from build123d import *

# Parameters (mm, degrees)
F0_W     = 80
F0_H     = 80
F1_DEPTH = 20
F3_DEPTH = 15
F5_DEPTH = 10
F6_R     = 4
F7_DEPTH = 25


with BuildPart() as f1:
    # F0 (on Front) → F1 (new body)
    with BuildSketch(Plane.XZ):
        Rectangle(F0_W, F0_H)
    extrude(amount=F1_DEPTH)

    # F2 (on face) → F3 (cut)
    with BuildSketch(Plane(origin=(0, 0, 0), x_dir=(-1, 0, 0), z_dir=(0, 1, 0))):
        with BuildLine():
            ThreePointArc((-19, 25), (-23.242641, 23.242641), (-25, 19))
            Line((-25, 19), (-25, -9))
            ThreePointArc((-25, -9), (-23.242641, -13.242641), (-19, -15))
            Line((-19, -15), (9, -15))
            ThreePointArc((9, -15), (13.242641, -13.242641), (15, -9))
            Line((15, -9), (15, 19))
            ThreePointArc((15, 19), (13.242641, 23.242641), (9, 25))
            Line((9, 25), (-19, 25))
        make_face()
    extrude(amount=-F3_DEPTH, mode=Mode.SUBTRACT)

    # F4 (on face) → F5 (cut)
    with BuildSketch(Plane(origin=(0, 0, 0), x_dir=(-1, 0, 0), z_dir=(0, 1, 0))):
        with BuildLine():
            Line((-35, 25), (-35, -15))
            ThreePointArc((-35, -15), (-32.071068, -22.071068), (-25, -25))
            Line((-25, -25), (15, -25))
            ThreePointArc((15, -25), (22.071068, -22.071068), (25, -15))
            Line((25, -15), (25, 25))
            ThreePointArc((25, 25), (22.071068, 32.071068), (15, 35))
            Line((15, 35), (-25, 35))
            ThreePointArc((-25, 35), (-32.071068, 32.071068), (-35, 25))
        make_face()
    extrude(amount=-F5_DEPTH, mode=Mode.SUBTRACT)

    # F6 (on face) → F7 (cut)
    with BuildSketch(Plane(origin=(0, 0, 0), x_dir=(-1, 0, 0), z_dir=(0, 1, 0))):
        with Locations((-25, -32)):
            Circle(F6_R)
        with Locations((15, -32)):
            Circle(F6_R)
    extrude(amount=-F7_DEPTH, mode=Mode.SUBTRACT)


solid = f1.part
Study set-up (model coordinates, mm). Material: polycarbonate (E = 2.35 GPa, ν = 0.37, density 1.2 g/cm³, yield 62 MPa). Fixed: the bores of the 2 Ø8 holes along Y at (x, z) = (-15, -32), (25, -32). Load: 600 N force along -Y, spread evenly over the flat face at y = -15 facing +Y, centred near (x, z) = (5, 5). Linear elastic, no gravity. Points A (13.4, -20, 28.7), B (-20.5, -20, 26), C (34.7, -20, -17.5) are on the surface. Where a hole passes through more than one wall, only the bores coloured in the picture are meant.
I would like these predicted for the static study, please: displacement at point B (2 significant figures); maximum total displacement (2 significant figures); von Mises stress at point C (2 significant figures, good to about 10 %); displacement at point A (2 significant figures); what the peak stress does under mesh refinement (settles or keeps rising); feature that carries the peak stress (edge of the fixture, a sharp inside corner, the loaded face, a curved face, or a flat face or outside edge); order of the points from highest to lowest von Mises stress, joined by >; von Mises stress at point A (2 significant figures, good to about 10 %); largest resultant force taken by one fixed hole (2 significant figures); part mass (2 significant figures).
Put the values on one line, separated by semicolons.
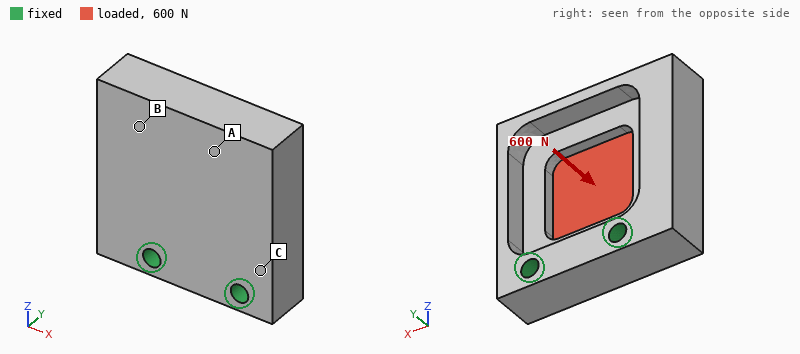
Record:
0.52 mm; 0.78 mm; 6.4 MPa; 0.66 mm; keeps rising; edge of the fixture; C > A > B; 3.6 MPa; 310 N; 100 g
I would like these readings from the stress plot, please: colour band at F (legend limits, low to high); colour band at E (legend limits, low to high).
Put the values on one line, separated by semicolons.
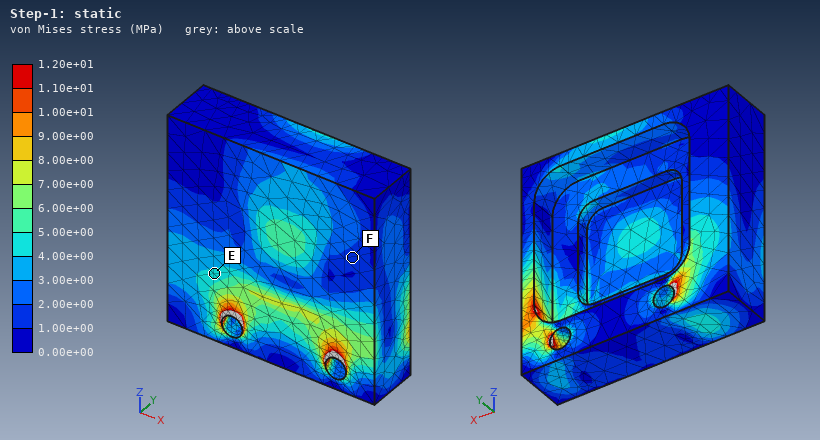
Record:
1.00e+00 to 2.00e+00 MPa; 4.00e+00 to 5.00e+00 MPa
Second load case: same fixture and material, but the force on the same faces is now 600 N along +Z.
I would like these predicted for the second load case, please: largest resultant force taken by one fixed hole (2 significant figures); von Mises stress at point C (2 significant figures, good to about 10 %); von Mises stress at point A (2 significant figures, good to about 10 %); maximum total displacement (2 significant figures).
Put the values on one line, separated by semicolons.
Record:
310 N; 0.58 MPa; 0.71 MPa; 30 µm
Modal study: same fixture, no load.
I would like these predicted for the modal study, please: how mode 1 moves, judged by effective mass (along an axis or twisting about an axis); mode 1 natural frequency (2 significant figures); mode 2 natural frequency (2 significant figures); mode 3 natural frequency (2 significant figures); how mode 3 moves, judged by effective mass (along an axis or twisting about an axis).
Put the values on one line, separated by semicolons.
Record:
along Y; 570 Hz; 860 Hz; 1500 Hz; along X
